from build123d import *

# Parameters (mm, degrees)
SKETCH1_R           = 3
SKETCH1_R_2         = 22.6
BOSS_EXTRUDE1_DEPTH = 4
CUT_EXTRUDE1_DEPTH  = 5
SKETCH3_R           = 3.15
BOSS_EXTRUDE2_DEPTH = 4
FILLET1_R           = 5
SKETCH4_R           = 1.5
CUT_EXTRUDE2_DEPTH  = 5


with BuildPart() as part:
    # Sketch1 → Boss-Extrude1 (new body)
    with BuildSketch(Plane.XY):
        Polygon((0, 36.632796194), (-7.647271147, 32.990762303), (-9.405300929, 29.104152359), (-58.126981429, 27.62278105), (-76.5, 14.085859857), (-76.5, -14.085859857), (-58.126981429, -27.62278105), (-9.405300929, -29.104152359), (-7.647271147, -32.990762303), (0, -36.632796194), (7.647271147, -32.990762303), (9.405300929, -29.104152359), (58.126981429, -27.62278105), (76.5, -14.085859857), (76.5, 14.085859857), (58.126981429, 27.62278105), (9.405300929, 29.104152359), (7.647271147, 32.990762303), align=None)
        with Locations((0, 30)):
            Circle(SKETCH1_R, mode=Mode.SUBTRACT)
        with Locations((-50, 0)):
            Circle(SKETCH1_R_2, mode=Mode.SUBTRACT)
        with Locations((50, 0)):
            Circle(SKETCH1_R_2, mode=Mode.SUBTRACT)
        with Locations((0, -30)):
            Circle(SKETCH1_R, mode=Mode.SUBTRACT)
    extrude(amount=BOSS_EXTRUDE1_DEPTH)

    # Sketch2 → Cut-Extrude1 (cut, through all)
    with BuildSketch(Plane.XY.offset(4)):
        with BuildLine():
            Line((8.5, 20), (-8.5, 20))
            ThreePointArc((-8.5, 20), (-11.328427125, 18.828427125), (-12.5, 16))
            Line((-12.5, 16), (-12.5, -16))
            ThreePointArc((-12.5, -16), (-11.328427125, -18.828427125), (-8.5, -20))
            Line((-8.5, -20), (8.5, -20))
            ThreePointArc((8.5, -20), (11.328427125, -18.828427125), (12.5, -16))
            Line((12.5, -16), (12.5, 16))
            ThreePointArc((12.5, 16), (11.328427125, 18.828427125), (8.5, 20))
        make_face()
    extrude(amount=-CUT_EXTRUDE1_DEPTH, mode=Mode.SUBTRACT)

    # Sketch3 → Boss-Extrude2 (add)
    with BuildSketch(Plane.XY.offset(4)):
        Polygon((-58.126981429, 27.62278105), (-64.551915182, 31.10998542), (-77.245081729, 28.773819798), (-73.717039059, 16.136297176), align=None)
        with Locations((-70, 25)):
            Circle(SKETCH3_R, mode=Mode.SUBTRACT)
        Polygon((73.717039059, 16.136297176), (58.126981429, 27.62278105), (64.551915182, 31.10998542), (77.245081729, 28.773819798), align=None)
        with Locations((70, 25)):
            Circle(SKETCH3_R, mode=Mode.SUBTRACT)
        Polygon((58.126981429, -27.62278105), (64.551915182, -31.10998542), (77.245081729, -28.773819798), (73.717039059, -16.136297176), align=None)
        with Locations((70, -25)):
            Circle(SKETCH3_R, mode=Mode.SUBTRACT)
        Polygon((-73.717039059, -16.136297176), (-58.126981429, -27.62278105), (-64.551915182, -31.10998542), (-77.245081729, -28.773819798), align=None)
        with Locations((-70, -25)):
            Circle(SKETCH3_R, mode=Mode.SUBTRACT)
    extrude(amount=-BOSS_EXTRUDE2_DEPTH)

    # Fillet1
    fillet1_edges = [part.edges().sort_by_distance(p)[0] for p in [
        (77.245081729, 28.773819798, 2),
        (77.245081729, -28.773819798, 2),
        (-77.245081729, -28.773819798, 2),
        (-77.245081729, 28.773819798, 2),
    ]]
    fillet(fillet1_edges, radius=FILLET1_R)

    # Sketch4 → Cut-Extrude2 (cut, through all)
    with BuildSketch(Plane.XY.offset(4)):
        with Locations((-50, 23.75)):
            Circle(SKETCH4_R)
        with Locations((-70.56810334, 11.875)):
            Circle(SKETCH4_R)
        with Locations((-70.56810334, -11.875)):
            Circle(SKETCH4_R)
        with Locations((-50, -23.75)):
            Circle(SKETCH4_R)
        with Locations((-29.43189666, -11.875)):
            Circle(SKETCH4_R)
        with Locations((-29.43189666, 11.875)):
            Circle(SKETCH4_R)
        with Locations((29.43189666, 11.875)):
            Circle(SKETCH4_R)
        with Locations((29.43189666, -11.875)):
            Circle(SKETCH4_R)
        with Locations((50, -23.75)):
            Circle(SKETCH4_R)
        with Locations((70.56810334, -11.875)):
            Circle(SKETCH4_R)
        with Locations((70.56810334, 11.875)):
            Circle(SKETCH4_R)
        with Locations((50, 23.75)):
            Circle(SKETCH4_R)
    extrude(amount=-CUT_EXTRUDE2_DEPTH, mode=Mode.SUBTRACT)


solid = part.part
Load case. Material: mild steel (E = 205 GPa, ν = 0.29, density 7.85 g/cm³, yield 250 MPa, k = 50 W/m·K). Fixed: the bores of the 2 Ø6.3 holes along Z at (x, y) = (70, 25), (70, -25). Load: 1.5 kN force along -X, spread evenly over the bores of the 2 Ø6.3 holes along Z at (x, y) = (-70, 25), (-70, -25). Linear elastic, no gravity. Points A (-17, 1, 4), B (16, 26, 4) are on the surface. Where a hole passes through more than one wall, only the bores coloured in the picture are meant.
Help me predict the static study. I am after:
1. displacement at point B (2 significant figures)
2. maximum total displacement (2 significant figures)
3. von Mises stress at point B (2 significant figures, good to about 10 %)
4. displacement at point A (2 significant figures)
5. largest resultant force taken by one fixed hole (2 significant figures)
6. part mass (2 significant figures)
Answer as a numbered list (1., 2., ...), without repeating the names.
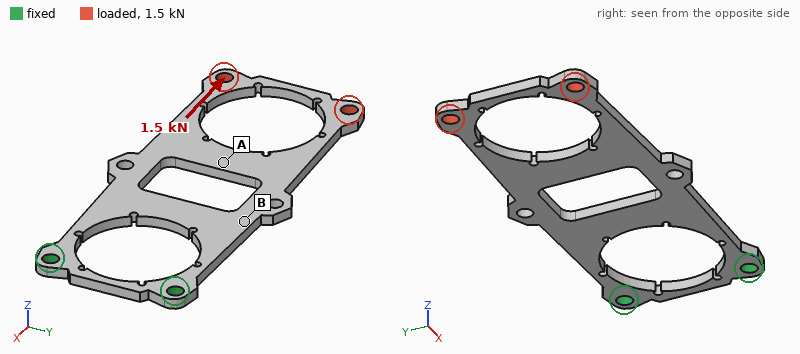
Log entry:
1. 9.3 µm
2. 28 µm
3. 20 MPa
4. 12 µm
5. 750 N
6. 140 g
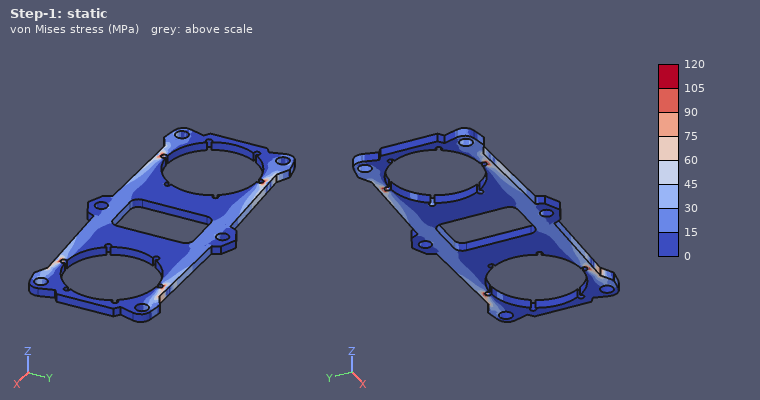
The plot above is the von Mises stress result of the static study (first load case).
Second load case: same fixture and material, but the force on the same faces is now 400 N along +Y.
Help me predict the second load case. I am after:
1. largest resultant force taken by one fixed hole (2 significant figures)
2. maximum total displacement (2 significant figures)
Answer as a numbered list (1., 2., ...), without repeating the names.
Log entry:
1. 950 N
2. 0.18 mm
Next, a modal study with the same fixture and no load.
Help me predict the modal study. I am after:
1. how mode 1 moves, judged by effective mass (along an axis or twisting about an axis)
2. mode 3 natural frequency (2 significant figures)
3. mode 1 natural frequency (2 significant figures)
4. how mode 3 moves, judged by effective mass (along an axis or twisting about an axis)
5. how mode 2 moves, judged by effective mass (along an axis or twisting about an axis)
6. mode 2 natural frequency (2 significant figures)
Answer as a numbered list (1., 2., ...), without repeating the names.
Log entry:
1. along Z
2. 730 Hz
3. 120 Hz
4. along Z
5. twisting about X
6. 610 Hz
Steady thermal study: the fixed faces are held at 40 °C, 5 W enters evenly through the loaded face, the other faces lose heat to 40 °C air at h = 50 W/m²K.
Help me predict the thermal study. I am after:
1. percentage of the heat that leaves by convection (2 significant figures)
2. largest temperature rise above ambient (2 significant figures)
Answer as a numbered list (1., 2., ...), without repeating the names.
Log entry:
1. 99 %
2. 39 K
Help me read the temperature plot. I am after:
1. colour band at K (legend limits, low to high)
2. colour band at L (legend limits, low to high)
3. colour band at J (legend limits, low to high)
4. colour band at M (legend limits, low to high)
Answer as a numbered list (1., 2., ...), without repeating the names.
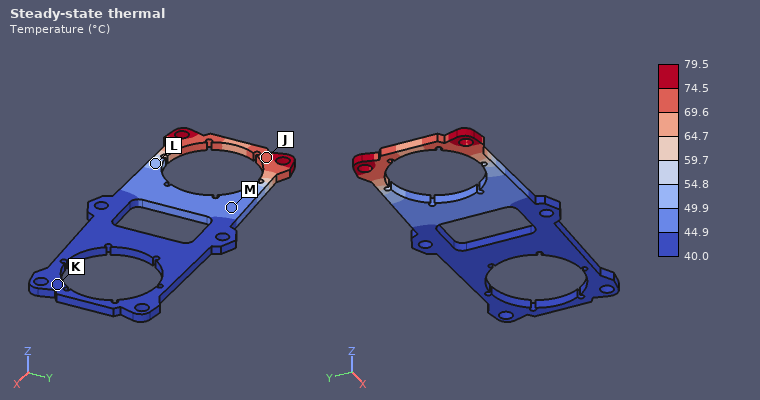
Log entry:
1. 40.0 to 44.9 °C
2. 49.9 to 54.8 °C
3. 69.6 to 74.5 °C
4. 44.9 to 49.9 °C
